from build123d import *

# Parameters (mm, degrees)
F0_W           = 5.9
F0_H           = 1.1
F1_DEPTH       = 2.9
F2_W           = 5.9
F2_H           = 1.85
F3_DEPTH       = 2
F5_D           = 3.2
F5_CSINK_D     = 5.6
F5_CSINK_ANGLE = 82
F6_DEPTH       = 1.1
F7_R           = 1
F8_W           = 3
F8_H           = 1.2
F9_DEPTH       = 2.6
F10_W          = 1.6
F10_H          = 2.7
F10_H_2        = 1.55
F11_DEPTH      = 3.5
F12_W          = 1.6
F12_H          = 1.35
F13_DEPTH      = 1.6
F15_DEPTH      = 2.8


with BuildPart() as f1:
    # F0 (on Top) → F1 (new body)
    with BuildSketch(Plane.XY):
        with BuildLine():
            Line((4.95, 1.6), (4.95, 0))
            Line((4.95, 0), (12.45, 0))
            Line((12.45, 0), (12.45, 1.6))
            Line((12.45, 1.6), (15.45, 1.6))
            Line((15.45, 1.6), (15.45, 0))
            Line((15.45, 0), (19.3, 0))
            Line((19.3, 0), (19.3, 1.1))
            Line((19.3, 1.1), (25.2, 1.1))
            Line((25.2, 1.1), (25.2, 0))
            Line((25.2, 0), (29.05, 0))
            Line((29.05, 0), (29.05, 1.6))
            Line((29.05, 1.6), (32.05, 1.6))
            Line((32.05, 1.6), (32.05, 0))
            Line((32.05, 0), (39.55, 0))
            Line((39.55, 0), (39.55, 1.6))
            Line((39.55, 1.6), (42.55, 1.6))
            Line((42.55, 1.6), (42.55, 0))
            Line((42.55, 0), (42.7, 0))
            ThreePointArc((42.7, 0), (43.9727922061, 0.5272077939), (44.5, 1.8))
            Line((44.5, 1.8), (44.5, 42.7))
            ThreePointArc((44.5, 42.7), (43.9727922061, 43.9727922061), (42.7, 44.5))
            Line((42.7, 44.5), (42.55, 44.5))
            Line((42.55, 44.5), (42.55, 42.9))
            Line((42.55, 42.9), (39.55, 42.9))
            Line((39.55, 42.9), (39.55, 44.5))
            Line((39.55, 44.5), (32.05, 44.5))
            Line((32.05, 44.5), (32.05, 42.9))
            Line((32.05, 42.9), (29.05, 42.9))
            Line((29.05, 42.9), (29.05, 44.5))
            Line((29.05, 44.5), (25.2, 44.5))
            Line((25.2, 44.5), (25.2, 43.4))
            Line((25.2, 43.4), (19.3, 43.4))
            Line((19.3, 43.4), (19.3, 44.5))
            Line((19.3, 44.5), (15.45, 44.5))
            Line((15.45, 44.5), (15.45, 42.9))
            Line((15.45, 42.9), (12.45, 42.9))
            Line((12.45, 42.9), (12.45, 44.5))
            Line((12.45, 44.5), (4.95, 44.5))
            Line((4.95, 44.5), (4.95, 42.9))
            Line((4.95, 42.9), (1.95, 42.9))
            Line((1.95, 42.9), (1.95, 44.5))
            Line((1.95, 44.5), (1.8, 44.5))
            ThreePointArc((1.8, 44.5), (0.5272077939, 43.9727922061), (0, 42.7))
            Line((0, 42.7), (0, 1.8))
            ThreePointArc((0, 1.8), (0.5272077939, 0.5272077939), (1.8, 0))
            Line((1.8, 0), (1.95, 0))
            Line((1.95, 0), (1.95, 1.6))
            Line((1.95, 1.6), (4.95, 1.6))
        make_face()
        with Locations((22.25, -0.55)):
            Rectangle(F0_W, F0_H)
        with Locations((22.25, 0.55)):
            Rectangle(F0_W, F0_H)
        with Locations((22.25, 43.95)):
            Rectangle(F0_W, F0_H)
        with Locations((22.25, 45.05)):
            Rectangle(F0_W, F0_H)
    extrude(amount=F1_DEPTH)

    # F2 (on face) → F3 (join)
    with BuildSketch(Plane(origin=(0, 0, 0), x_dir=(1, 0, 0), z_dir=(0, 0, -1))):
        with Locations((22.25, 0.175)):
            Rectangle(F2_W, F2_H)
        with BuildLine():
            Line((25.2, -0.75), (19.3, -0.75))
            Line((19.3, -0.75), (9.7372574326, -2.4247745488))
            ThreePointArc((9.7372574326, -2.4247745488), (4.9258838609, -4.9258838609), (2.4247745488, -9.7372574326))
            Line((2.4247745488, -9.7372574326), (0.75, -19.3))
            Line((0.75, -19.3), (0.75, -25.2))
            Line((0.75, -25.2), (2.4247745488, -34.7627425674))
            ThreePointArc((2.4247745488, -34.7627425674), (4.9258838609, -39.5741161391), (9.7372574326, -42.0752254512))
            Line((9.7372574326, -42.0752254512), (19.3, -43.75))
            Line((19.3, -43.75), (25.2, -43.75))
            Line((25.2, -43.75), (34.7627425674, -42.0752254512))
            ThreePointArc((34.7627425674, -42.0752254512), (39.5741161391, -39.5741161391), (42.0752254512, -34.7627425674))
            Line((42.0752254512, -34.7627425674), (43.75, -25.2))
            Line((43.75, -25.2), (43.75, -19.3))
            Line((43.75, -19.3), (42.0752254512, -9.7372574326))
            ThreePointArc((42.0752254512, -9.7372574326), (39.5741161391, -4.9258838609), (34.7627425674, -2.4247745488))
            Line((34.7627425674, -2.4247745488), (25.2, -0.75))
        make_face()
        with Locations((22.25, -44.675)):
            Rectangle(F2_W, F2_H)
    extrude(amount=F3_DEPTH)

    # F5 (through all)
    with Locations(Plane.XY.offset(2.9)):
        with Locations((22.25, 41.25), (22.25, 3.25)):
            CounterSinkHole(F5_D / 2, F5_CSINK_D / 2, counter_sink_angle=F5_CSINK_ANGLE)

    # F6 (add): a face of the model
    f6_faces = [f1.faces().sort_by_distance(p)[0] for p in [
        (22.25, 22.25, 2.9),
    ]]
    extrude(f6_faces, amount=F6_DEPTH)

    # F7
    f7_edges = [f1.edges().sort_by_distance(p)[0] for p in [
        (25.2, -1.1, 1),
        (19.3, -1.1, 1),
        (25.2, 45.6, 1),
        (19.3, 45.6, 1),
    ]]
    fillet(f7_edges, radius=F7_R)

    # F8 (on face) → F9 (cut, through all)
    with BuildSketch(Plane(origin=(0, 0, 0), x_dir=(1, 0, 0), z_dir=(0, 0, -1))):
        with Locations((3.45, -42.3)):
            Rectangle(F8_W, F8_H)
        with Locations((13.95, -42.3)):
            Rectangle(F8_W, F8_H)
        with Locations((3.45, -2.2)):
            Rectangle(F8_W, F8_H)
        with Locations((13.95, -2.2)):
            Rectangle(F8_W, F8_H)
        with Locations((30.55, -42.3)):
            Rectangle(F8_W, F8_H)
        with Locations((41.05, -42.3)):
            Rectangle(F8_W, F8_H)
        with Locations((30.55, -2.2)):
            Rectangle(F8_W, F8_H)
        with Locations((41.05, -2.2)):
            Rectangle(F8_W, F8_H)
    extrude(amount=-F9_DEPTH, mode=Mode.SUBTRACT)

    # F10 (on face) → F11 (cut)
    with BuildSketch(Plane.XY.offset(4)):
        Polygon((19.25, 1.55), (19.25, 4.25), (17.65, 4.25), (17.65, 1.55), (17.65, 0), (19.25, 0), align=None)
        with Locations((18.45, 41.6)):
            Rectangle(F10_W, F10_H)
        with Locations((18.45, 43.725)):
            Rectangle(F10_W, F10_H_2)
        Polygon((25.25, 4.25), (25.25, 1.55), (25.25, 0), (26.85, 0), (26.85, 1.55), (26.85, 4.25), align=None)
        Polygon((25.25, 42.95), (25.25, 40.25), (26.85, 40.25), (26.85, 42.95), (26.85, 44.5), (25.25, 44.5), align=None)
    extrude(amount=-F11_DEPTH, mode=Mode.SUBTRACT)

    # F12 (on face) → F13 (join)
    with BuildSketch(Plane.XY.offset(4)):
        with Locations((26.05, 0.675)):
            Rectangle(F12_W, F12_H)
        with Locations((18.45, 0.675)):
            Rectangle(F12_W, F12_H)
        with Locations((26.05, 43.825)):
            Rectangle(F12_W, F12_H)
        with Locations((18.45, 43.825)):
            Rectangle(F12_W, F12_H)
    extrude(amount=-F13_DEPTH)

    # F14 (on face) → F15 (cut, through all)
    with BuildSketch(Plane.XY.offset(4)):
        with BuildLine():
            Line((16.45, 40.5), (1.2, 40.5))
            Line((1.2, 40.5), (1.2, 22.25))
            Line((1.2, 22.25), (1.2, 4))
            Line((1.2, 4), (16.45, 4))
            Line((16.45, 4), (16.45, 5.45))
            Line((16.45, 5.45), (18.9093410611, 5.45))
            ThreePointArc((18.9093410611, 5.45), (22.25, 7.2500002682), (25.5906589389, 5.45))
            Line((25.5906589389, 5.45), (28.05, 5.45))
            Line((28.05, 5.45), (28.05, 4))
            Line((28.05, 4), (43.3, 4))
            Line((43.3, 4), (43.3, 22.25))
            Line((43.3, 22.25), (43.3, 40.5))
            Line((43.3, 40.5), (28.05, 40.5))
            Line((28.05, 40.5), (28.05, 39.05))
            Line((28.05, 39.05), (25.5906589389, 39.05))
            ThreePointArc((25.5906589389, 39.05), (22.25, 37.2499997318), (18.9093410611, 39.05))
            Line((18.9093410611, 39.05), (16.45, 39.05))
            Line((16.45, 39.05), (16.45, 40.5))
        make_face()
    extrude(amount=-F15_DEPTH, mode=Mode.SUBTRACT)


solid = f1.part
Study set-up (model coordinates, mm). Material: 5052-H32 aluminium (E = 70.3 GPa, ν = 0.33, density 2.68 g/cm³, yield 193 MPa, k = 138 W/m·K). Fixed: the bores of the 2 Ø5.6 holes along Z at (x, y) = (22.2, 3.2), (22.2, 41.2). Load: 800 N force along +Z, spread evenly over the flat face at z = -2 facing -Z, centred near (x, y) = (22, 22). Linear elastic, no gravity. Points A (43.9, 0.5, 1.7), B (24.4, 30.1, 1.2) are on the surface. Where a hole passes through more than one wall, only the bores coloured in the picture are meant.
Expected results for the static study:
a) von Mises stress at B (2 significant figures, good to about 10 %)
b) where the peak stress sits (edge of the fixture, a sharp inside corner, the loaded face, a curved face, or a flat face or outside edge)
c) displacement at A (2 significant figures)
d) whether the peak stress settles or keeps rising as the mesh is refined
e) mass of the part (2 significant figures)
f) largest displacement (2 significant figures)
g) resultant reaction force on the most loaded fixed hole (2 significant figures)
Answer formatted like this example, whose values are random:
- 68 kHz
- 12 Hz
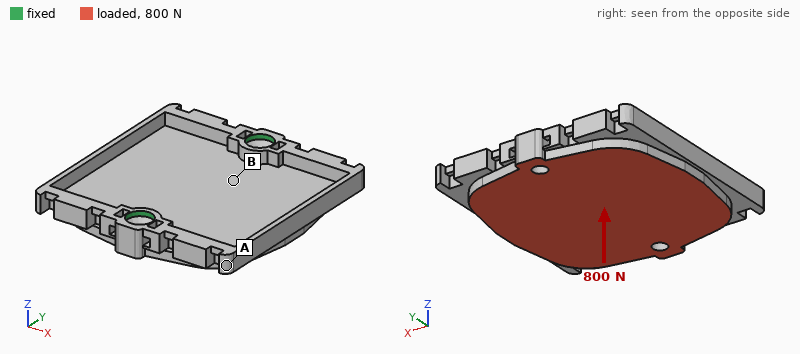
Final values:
- 19 MPa
- edge of the fixture
- 23 µm
- keeps rising
- 18 g
- 47 µm
- 470 N
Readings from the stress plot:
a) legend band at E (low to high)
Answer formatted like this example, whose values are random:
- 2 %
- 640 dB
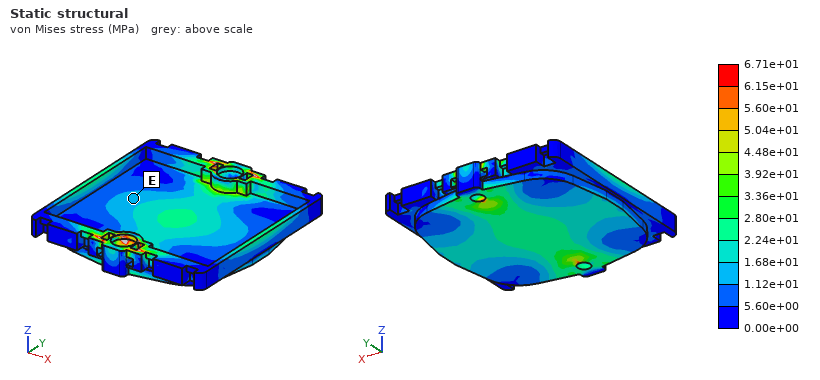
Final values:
- 1.12e+01 to 1.68e+01 MPa
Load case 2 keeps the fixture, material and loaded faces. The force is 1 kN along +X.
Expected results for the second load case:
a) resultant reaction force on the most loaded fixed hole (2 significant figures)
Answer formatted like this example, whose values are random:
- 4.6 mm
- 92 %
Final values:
- 500 N
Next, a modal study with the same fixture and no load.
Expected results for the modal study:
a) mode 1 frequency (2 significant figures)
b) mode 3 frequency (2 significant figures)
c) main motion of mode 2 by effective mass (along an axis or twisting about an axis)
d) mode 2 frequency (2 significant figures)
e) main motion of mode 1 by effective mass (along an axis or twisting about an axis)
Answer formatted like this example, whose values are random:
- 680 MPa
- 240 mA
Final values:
- 4300 Hz
- 8300 Hz
- along Z
- 6300 Hz
- twisting about Y
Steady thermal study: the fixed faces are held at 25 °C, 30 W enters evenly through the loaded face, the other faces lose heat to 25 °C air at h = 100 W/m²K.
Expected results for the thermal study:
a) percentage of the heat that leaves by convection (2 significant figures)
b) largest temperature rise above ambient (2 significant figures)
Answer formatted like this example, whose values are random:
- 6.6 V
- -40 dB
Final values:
- 18 %
- 18 K
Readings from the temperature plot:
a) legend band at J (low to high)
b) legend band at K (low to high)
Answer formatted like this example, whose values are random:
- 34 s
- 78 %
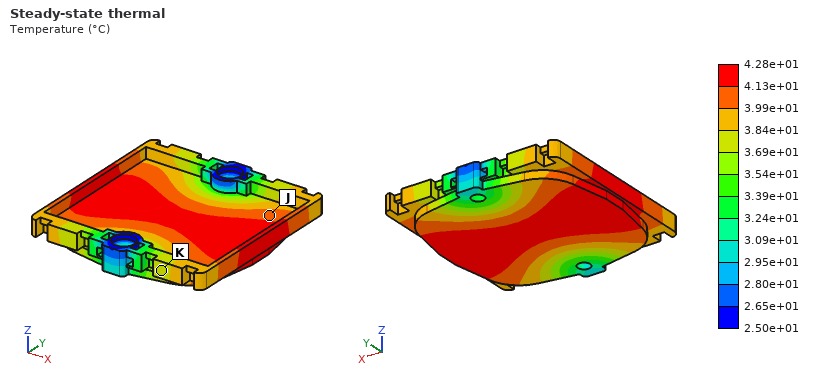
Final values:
- 3.99e+01 to 4.13e+01 °C
- 3.69e+01 to 3.84e+01 °C
